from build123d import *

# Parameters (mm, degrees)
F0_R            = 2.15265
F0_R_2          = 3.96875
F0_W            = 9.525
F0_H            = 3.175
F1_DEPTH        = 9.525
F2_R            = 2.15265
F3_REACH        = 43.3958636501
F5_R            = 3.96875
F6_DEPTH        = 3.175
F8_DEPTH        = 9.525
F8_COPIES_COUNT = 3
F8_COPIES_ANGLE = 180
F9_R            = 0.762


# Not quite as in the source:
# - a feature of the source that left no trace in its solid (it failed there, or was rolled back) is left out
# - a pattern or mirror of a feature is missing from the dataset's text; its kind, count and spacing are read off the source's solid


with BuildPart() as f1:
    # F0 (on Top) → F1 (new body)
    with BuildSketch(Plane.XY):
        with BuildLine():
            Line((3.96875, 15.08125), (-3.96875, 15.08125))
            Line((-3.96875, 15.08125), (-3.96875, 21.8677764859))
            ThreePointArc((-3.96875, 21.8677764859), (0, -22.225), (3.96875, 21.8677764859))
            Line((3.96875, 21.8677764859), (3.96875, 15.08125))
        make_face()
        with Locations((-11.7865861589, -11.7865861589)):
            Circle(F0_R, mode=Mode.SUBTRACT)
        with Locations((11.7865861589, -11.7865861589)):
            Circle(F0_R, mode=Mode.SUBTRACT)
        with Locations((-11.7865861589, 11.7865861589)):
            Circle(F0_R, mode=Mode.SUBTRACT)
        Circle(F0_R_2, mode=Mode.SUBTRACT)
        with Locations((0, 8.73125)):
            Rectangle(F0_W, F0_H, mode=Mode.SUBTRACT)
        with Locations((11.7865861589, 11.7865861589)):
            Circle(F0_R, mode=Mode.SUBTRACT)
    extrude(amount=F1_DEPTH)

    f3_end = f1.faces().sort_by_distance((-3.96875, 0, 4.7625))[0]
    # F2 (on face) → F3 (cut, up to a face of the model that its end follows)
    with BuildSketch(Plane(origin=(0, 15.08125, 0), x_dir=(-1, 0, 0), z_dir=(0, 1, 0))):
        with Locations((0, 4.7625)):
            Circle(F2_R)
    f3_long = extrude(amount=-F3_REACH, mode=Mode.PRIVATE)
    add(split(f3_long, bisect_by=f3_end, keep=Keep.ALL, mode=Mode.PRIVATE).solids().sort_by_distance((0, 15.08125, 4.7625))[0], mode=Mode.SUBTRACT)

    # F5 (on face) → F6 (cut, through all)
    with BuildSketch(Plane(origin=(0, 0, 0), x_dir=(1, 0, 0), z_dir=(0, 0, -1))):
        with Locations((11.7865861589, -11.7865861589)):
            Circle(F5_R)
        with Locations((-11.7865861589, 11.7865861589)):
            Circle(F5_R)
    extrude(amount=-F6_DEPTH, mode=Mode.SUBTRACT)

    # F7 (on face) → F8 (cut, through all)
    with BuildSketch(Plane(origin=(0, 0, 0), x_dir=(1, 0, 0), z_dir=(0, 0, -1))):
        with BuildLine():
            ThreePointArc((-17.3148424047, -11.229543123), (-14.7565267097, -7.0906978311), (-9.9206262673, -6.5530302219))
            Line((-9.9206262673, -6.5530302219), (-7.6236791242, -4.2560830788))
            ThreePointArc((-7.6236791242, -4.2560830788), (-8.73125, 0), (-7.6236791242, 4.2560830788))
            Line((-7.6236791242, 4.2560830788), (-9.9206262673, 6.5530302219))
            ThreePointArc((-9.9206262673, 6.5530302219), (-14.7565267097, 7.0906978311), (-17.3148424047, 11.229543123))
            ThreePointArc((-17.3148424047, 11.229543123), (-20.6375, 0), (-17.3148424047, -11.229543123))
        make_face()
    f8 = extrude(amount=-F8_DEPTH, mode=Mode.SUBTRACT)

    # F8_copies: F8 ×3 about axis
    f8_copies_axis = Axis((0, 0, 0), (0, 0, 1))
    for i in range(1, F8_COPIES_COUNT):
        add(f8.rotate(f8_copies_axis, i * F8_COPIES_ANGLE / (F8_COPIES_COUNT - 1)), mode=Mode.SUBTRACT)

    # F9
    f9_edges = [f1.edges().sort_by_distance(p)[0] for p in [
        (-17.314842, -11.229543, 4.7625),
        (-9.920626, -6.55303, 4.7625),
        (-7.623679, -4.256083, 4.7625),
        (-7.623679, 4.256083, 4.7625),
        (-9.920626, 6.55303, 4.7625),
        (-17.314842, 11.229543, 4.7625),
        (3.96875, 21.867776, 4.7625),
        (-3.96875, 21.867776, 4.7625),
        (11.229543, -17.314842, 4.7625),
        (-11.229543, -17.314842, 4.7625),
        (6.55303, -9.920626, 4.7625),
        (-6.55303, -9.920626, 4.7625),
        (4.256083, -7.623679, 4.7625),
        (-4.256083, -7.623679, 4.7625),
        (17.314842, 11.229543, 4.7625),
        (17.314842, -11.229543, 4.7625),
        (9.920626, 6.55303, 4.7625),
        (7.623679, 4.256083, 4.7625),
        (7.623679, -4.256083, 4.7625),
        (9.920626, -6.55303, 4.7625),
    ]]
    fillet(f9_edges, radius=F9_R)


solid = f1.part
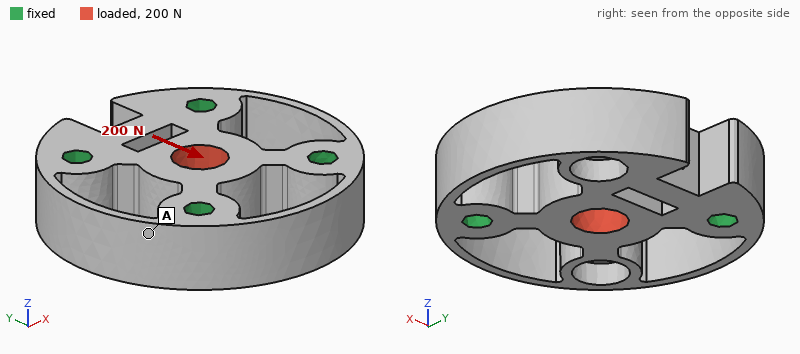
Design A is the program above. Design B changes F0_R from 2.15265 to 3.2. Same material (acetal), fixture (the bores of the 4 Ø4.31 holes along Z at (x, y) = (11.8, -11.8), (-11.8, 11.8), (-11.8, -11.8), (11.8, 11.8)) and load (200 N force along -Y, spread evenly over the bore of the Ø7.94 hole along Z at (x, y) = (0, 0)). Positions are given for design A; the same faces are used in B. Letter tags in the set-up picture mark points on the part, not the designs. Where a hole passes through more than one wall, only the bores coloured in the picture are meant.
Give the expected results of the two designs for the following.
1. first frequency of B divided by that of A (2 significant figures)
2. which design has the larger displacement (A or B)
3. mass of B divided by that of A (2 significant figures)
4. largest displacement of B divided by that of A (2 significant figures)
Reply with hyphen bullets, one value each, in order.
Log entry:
- 1.1
- A
- 0.93
- 0.90
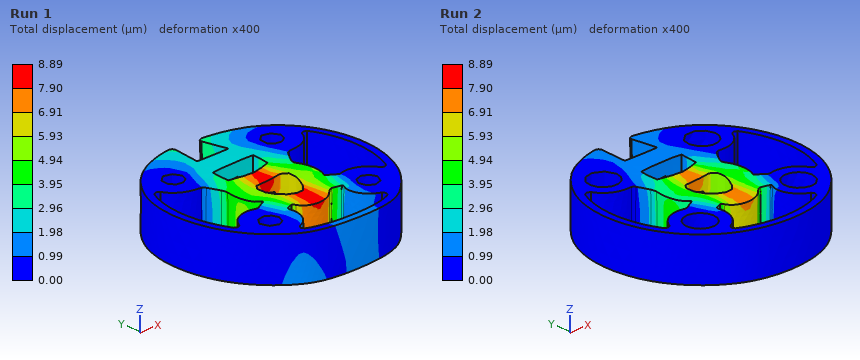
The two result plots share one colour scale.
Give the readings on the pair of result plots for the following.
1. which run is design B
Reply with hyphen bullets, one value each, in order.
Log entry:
- Run 2
